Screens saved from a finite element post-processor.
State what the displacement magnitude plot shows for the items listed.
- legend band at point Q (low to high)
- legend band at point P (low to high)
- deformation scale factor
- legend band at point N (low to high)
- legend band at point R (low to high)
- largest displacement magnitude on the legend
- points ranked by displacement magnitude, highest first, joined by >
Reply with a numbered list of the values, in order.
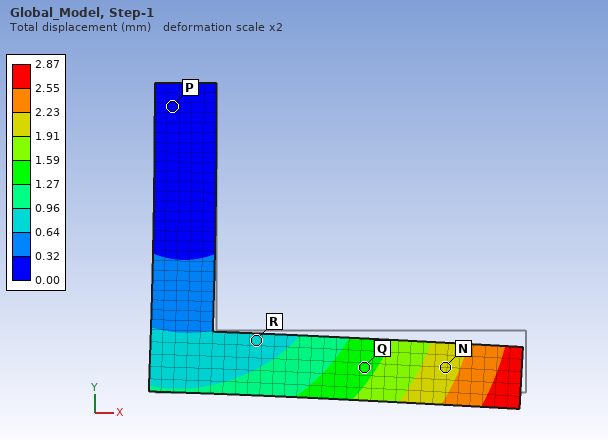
1. 1.27 to 1.59 mm
2. 0.00 to 0.32 mm
3. 2
4. 1.91 to 2.23 mm
5. 0.64 to 0.96 mm
6. 2.87 mm
7. N > Q > R > P
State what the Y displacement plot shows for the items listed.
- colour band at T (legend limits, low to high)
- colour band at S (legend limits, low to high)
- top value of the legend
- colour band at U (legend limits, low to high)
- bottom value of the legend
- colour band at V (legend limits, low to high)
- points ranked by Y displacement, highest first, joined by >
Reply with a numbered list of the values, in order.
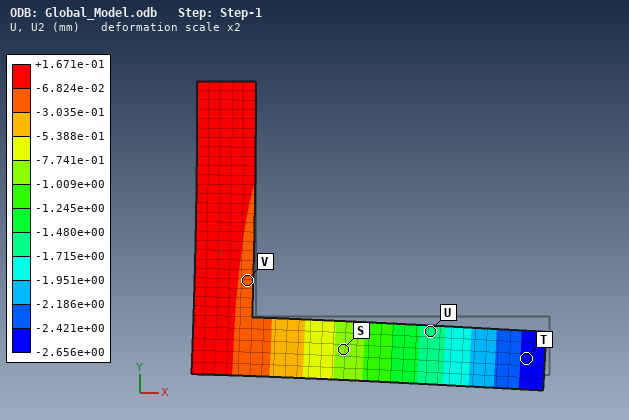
1. -2.656e+00 to -2.421e+00 mm
2. -1.009e+00 to -7.741e-01 mm
3. +1.671e-01 mm
4. -1.715e+00 to -1.480e+00 mm
5. -2.656e+00 mm
6. -3.035e-01 to -6.824e-02 mm
7. V > S > U > T
